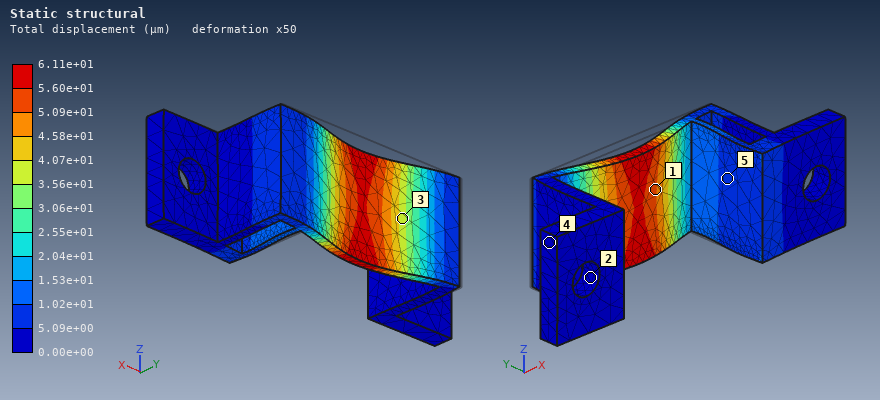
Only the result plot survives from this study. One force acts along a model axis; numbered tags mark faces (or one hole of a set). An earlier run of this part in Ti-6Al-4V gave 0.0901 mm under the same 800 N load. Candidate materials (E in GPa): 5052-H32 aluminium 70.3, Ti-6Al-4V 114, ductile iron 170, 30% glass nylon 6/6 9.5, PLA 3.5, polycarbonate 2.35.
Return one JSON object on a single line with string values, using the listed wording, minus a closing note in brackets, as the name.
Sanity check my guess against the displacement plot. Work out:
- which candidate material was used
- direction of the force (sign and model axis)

{"which candidate material was used": "ductile iron", "direction of the force": "-Y"}
